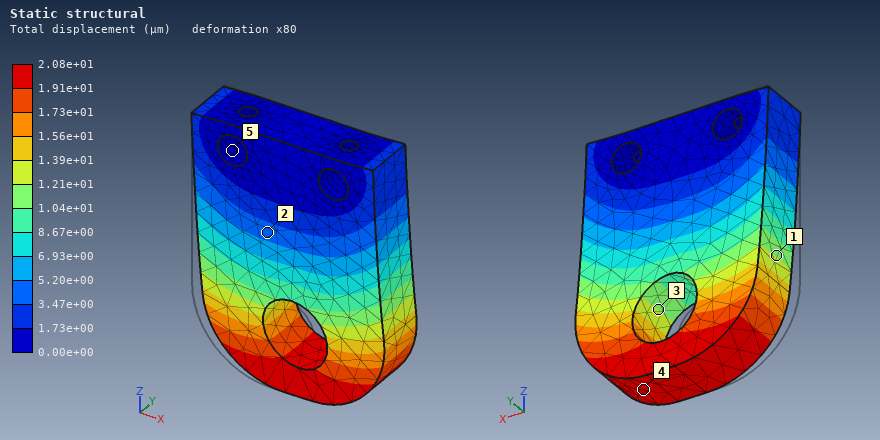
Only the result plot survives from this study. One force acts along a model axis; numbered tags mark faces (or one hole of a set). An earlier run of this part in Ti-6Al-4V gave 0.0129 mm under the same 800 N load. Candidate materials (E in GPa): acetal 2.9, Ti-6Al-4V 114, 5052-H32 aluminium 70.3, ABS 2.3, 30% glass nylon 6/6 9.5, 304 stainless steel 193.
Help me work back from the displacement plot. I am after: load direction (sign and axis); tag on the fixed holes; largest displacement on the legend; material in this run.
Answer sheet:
+X
5
2.08e+01 µm
5052-H32 aluminium
